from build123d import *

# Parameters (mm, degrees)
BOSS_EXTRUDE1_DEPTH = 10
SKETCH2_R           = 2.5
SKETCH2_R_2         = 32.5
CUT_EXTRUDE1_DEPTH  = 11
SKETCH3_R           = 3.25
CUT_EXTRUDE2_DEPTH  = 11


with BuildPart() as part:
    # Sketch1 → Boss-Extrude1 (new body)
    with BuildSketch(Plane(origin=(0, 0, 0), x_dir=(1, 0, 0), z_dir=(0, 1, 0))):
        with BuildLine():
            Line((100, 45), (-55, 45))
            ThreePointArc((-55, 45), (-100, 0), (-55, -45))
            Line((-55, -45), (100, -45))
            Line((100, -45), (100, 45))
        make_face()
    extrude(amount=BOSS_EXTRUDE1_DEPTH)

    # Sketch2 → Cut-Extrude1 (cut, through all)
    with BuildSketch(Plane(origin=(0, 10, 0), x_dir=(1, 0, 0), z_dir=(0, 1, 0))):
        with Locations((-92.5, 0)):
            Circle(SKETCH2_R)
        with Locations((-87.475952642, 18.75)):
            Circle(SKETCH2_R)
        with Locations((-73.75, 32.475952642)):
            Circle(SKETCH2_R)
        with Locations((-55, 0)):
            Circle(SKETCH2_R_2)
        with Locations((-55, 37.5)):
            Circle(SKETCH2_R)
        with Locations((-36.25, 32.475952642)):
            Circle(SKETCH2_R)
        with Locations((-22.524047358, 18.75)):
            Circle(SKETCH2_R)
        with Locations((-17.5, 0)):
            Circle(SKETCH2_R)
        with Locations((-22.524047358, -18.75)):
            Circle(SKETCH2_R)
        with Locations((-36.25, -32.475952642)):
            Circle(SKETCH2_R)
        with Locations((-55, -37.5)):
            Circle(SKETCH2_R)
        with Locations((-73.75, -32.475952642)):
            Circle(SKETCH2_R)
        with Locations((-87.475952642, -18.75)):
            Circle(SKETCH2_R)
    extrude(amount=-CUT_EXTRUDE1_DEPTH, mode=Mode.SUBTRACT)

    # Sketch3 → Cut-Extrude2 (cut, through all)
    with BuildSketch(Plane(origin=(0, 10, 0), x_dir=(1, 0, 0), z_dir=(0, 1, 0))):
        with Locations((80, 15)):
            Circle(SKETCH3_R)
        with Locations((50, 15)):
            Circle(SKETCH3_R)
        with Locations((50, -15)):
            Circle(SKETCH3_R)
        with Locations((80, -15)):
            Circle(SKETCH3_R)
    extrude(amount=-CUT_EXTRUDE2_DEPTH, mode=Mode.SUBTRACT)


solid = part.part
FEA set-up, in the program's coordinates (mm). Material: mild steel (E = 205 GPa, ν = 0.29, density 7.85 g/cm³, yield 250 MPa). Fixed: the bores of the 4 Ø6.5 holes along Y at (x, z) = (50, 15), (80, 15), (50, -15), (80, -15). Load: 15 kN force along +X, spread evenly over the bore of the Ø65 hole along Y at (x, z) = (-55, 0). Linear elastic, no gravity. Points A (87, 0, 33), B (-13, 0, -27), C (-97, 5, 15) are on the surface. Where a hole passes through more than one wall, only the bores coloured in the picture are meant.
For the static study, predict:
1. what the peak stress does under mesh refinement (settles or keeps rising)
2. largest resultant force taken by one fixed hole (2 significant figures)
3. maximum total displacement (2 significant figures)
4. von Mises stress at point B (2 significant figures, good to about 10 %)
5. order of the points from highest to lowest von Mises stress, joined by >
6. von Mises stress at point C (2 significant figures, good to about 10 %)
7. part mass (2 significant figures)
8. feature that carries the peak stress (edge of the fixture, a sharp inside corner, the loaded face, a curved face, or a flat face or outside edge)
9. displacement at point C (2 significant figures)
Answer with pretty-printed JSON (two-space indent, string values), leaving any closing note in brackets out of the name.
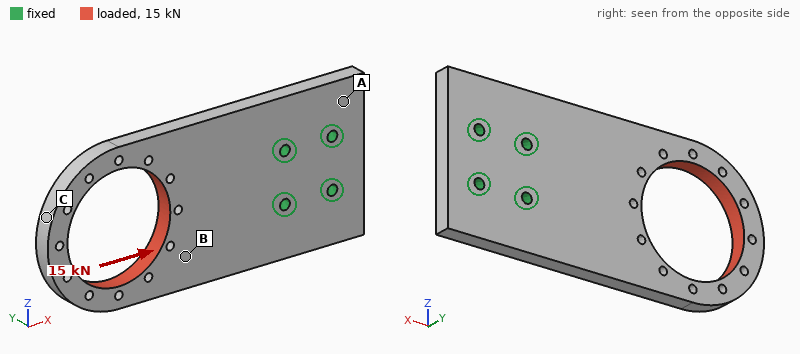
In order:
{
  "what the peak stress does under mesh refinement": "keeps rising",
  "largest resultant force taken by one fixed hole": "5.7 kN",
  "maximum total displacement": "48 µm",
  "von Mises stress at point B": "22 MPa",
  "order of the points from highest to lowest von Mises stress, joined by >": "C > B > A",
  "von Mises stress at point C": "56 MPa",
  "part mass": "1.1 kg",
  "feature that carries the peak stress": "a sharp inside corner",
  "displacement at point C": "41 µm"
}
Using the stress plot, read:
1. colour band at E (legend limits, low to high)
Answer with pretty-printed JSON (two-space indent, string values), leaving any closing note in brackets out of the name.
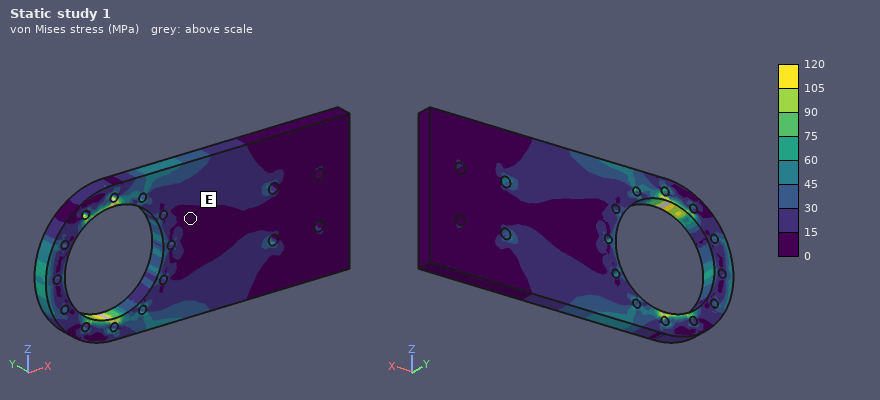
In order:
{
  "colour band at E": "0 to 15 MPa"
}
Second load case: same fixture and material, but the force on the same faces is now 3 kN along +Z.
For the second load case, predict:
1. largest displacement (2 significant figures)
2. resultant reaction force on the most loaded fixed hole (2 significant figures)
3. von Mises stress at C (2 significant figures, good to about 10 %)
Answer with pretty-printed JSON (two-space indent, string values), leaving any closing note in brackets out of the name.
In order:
{
  "largest displacement": "68 µm",
  "resultant reaction force on the most loaded fixed hole": "5.3 kN",
  "von Mises stress at C": "15 MPa"
}
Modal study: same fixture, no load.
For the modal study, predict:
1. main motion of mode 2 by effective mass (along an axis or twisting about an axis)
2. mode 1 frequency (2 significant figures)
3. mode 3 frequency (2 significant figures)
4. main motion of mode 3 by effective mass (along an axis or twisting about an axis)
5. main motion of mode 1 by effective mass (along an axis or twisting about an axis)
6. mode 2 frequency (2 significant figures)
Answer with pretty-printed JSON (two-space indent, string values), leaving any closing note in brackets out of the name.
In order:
{
  "main motion of mode 2 by effective mass": "twisting about X",
  "mode 1 frequency": "540 Hz",
  "mode 3 frequency": "1900 Hz",
  "main motion of mode 3 by effective mass": "along Y",
  "main motion of mode 1 by effective mass": "along Y",
  "mode 2 frequency": "1400 Hz"
}
